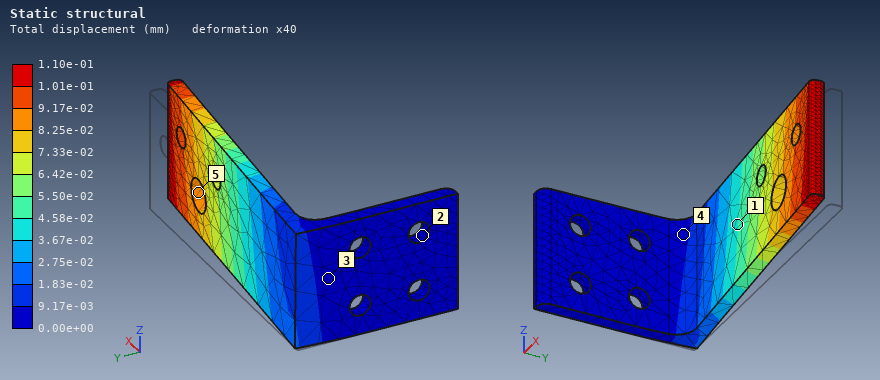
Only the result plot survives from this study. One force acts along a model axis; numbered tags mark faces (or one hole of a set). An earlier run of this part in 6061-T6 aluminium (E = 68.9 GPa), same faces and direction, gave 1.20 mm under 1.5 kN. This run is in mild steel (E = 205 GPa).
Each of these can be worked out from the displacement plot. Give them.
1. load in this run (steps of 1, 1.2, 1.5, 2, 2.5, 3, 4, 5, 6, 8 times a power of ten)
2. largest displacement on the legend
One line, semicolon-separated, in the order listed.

400 N; 1.10e-01 mm
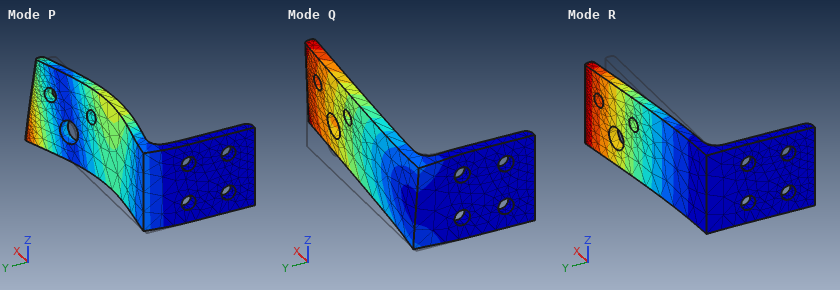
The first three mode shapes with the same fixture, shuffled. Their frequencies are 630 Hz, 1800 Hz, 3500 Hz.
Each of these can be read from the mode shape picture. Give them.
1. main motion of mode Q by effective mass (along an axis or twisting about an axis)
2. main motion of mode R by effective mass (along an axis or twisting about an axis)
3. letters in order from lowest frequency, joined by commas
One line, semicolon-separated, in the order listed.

along Z; along Y; R, Q, P
